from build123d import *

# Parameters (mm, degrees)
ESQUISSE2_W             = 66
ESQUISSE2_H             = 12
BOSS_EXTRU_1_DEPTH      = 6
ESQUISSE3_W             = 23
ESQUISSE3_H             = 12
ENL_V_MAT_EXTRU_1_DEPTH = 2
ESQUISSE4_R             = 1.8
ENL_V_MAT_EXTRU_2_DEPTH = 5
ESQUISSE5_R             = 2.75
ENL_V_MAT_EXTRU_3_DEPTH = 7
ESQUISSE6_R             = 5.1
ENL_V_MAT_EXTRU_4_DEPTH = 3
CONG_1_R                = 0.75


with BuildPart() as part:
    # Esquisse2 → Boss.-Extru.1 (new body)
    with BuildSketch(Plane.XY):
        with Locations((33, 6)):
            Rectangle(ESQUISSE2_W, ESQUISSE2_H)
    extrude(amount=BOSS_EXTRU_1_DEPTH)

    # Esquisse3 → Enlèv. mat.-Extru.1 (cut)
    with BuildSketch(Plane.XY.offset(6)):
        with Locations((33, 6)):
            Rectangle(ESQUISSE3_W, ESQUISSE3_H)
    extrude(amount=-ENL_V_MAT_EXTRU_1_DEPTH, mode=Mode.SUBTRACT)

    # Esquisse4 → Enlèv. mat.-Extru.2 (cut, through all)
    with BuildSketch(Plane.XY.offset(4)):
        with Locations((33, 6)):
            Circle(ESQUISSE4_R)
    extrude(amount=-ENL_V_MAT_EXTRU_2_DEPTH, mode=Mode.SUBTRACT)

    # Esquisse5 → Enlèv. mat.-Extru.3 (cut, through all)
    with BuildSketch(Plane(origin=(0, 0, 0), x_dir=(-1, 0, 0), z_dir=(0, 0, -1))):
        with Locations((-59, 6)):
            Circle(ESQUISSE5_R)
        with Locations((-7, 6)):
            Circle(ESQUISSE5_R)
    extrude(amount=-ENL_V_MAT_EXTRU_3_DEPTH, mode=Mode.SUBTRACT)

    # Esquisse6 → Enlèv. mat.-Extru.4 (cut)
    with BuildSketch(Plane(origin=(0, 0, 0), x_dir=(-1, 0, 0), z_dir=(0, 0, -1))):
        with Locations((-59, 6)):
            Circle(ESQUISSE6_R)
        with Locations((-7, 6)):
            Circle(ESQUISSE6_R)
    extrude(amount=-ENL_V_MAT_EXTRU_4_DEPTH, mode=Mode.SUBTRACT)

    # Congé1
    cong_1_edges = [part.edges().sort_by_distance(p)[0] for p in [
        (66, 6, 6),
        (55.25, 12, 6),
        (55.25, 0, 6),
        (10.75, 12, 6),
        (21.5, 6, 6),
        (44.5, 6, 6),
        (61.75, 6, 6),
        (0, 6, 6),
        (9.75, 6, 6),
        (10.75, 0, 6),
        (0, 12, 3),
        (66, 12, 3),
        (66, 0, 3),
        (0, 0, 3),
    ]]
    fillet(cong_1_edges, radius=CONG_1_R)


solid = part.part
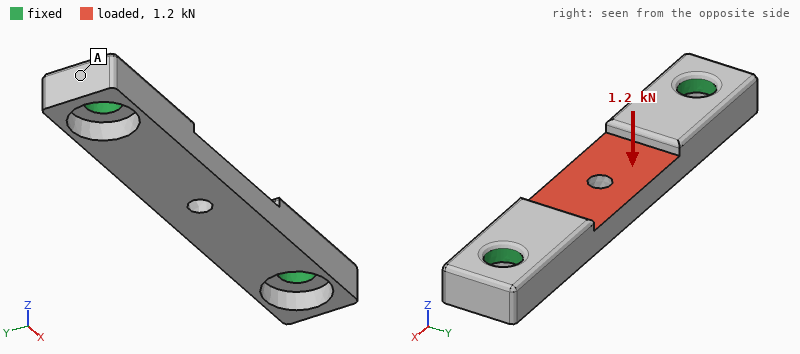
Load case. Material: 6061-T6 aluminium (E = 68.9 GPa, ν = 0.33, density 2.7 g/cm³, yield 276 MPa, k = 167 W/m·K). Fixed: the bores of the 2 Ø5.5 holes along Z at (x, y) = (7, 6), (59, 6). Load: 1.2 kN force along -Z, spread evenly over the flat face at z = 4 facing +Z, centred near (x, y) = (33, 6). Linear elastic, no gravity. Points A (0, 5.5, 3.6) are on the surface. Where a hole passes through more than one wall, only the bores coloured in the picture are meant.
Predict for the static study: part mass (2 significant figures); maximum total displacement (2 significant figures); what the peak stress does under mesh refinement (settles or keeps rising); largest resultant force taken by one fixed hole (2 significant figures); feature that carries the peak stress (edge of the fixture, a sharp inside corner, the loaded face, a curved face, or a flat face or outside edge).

9.5 g
0.12 mm
keeps rising
1.6 kN
edge of the fixture
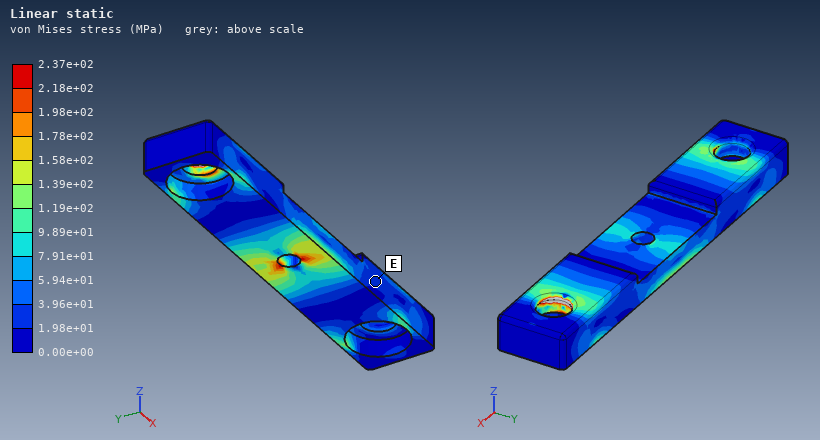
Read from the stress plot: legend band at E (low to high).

1.98e+01 to 3.96e+01 MPa
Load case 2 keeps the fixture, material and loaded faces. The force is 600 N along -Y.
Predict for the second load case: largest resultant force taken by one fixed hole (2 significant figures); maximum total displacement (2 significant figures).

300 N
18 µm
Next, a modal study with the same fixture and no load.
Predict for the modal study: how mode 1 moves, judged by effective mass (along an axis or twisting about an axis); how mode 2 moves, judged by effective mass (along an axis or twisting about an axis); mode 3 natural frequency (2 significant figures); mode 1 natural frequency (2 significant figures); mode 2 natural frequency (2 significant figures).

along Z
along Y
19 kHz
9200 Hz
15 kHz
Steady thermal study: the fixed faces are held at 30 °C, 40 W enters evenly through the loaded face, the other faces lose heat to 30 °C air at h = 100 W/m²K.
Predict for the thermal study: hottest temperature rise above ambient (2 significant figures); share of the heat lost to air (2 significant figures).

41 K
8.6 %
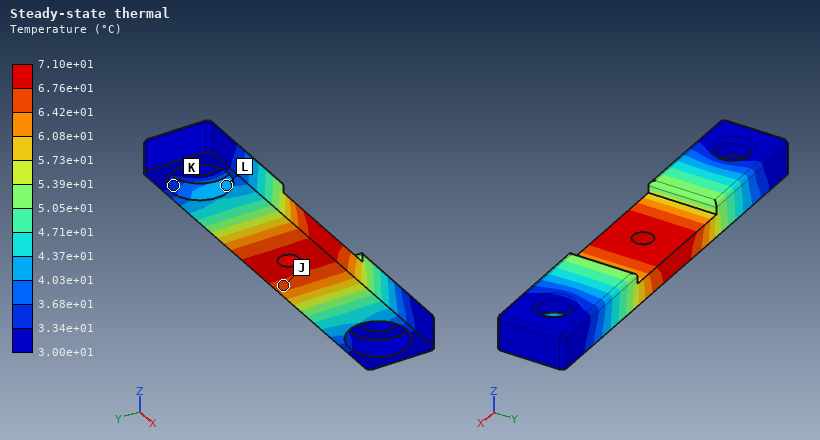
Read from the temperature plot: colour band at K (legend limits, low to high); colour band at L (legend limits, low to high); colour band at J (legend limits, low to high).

3.34e+01 to 3.68e+01 °C
4.03e+01 to 4.37e+01 °C
6.42e+01 to 6.76e+01 °C
